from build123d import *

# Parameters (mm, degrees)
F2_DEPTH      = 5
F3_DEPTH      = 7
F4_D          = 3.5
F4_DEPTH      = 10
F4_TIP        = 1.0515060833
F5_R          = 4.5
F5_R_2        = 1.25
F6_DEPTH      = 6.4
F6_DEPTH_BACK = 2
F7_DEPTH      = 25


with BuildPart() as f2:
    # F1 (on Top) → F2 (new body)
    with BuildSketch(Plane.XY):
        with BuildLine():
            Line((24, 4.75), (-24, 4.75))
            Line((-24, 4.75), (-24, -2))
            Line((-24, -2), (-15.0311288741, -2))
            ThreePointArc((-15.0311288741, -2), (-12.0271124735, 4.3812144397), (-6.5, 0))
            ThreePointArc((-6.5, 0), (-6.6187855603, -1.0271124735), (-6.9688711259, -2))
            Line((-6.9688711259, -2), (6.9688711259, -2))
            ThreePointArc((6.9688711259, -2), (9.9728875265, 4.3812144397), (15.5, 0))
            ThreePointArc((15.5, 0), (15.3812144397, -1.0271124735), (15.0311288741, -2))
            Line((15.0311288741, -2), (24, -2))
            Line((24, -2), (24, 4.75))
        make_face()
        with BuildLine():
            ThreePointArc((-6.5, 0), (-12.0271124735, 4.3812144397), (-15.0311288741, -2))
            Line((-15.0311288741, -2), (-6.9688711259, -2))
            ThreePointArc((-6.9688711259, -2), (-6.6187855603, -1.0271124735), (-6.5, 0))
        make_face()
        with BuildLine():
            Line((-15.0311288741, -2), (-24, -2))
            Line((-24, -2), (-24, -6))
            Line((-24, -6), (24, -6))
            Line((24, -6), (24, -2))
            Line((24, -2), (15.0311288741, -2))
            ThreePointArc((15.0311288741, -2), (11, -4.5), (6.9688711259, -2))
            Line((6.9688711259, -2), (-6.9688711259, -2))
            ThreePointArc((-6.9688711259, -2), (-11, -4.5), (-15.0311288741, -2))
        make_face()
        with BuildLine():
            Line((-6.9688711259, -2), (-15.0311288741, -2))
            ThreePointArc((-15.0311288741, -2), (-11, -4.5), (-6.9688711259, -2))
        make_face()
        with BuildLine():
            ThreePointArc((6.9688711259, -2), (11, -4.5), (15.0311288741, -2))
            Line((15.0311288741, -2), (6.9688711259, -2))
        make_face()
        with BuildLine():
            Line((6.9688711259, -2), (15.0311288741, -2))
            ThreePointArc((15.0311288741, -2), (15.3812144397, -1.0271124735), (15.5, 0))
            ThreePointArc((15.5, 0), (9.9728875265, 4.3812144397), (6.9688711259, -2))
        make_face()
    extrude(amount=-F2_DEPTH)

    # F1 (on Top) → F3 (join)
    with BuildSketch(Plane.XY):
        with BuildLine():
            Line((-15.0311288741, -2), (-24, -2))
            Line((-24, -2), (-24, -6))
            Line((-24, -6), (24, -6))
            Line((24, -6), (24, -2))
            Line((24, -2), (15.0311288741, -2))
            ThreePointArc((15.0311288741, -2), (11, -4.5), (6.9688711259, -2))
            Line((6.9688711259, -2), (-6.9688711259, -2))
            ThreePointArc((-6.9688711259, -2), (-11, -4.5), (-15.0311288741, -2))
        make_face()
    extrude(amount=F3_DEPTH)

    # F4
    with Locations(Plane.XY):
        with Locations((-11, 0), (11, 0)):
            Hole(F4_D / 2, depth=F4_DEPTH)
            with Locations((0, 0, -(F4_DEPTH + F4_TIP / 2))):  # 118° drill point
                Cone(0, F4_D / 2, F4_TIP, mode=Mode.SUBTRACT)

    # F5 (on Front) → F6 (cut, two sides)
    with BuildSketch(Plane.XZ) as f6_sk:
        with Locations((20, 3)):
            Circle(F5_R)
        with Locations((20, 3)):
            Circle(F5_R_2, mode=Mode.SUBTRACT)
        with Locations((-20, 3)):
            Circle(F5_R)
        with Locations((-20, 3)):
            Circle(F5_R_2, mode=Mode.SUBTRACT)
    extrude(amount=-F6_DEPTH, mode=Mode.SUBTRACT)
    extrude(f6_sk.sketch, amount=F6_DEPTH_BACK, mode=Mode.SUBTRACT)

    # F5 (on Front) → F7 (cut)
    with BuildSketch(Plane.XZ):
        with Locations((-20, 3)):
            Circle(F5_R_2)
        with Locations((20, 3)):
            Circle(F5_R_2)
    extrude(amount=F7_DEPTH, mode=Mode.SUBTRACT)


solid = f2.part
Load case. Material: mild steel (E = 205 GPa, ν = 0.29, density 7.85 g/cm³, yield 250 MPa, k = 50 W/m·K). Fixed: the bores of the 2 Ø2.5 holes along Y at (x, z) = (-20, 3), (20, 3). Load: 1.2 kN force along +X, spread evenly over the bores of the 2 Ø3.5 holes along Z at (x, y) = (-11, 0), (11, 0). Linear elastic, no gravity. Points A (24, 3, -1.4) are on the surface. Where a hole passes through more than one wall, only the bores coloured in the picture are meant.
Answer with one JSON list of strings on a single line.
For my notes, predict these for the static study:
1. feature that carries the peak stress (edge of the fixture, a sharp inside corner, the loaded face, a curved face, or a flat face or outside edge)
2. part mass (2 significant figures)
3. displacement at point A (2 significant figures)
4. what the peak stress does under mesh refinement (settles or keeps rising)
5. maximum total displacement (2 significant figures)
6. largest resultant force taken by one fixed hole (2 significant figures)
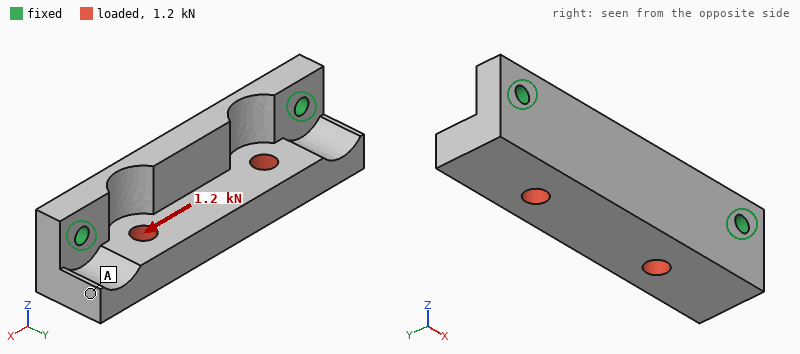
["edge of the fixture", "27 g", "1.8 µm", "keeps rising", "2.3 µm", "630 N"]
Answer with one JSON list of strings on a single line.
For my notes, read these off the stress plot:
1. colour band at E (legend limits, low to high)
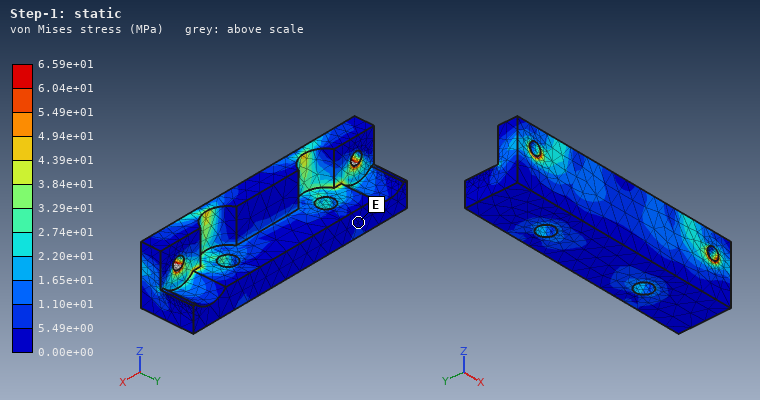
["0.00e+00 to 5.49e+00 MPa"]
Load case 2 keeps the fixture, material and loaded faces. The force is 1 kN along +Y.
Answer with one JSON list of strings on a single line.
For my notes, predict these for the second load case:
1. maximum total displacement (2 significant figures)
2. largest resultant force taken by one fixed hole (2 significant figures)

["14 µm", "520 N"]
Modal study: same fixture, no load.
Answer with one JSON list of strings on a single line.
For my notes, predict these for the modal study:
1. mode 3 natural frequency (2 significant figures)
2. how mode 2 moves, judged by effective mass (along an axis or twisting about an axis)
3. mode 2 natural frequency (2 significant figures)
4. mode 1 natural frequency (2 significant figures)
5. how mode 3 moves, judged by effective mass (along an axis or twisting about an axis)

["19 kHz", "along Y", "15 kHz", "10 kHz", "along Z"]
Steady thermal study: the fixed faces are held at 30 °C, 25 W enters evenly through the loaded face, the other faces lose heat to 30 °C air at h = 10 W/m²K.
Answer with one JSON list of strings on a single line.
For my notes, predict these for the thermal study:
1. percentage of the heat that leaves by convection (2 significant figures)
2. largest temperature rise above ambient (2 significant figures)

["3.4 %", "63 K"]
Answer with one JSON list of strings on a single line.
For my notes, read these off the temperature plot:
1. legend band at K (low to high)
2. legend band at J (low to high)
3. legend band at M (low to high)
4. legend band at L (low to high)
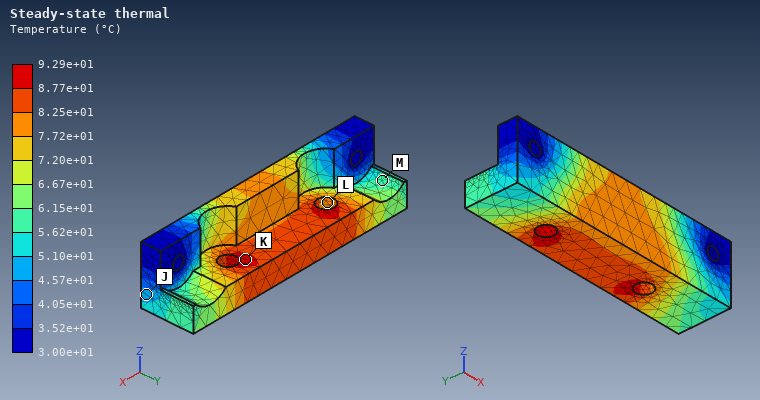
["8.77e+01 to 9.29e+01 °C", "4.57e+01 to 5.10e+01 °C", "5.62e+01 to 6.15e+01 °C", "7.72e+01 to 8.25e+01 °C"]
